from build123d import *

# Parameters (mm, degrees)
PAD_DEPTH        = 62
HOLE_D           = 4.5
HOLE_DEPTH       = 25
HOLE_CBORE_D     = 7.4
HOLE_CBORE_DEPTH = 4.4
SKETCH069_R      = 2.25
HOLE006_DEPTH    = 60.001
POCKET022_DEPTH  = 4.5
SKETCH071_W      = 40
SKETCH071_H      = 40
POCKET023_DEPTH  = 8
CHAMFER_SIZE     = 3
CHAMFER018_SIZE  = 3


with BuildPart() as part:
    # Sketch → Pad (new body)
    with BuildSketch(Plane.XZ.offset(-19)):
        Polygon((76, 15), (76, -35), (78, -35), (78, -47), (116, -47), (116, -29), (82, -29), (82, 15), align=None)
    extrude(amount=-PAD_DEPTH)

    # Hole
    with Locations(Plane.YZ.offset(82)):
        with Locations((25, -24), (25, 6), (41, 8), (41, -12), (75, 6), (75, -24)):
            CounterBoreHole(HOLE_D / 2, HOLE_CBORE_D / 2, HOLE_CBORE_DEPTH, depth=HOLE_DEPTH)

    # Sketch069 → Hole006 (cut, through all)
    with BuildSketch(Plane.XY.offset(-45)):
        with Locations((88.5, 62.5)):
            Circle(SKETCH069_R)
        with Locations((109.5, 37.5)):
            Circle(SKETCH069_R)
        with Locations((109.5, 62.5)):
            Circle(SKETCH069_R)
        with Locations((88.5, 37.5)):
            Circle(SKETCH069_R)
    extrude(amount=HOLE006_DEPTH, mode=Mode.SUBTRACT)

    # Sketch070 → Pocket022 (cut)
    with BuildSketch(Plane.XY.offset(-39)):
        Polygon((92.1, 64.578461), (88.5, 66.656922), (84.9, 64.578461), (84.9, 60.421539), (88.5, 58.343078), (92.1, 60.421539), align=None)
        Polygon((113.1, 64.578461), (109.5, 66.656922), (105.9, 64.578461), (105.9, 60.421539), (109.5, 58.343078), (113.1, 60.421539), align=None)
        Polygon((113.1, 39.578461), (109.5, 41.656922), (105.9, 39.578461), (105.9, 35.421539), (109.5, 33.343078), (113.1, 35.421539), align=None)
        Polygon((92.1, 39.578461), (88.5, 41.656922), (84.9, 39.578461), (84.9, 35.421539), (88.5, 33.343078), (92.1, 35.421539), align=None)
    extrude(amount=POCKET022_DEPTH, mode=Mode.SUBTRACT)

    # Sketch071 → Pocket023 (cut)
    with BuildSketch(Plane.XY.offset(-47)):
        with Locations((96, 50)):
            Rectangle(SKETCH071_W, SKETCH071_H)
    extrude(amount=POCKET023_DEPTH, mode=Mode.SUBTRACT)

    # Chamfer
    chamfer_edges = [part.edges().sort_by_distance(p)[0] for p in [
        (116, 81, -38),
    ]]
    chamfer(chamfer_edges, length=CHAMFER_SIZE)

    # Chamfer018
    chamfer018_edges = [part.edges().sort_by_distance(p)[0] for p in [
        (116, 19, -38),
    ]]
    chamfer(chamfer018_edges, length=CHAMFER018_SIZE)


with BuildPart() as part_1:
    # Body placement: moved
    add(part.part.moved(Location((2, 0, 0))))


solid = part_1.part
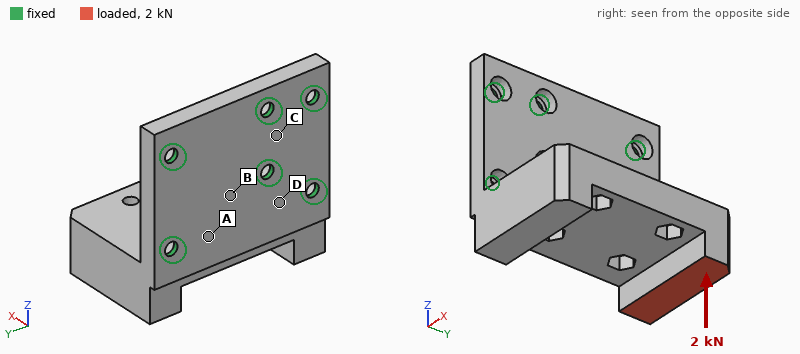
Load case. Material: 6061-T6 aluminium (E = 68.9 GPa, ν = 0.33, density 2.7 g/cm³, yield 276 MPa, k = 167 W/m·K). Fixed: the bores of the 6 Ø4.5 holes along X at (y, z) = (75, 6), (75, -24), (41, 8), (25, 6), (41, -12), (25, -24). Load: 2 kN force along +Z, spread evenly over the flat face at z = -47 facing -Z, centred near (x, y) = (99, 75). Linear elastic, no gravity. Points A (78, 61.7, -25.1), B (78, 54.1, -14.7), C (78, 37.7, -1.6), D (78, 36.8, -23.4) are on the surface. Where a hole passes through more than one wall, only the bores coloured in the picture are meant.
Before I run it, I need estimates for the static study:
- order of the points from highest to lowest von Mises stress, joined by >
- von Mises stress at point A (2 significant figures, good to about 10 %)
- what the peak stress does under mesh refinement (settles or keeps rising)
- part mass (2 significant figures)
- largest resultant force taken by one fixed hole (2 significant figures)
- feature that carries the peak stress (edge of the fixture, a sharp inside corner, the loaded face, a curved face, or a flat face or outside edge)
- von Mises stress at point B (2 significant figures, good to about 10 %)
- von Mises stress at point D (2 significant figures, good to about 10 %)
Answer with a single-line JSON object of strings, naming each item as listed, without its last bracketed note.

{"order of the points from highest to lowest von Mises stress, joined by >": "A > D > B > C", "von Mises stress at point A": "76 MPa", "what the peak stress does under mesh refinement": "keeps rising", "part mass": "120 g", "largest resultant force taken by one fixed hole": "1.6 kN", "feature that carries the peak stress": "edge of the fixture", "von Mises stress at point B": "29 MPa", "von Mises stress at point D": "55 MPa"}
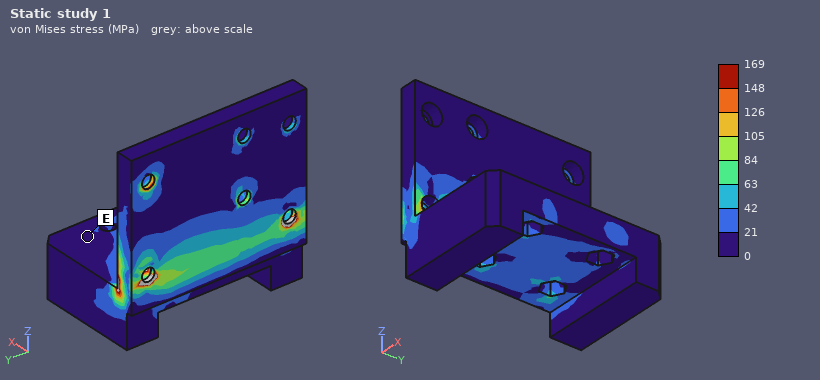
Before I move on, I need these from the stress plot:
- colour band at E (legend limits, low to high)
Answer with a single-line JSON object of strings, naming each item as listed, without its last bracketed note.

{"colour band at E": "0 to 21 MPa"}
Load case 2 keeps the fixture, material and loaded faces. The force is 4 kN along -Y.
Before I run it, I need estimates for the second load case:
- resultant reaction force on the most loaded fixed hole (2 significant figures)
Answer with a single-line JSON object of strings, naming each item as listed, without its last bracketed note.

{"resultant reaction force on the most loaded fixed hole": "2.8 kN"}
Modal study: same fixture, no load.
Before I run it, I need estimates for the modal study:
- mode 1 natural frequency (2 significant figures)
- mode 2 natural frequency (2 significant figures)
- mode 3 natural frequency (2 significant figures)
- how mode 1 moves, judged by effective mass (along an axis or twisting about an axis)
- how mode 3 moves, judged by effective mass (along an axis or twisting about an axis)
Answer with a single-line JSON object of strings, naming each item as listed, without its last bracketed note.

{"mode 1 natural frequency": "1700 Hz", "mode 2 natural frequency": "4300 Hz", "mode 3 natural frequency": "6600 Hz", "how mode 1 moves, judged by effective mass": "along Z", "how mode 3 moves, judged by effective mass": "along Y"}
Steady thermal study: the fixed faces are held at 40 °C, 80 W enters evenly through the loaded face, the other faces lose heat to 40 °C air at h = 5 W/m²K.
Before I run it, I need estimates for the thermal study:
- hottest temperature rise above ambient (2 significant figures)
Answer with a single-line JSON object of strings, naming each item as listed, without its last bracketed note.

{"hottest temperature rise above ambient": "63 K"}
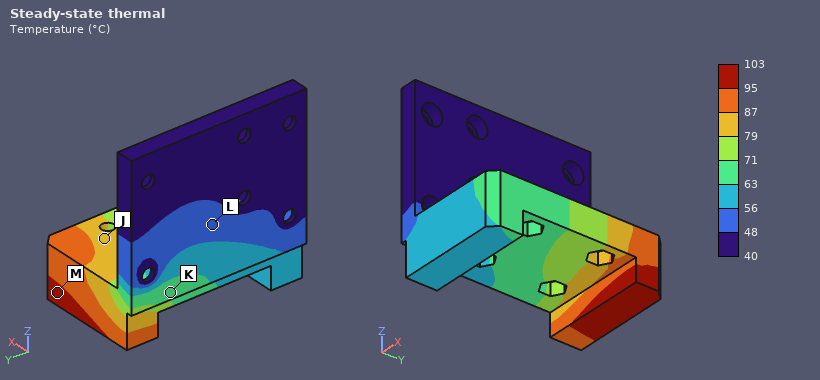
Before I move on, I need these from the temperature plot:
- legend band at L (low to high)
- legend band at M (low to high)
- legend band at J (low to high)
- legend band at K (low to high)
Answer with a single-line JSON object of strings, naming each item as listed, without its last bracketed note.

{"legend band at L": "48 to 56 °C", "legend band at M": "95 to 103 °C", "legend band at J": "79 to 87 °C", "legend band at K": "63 to 71 °C"}
